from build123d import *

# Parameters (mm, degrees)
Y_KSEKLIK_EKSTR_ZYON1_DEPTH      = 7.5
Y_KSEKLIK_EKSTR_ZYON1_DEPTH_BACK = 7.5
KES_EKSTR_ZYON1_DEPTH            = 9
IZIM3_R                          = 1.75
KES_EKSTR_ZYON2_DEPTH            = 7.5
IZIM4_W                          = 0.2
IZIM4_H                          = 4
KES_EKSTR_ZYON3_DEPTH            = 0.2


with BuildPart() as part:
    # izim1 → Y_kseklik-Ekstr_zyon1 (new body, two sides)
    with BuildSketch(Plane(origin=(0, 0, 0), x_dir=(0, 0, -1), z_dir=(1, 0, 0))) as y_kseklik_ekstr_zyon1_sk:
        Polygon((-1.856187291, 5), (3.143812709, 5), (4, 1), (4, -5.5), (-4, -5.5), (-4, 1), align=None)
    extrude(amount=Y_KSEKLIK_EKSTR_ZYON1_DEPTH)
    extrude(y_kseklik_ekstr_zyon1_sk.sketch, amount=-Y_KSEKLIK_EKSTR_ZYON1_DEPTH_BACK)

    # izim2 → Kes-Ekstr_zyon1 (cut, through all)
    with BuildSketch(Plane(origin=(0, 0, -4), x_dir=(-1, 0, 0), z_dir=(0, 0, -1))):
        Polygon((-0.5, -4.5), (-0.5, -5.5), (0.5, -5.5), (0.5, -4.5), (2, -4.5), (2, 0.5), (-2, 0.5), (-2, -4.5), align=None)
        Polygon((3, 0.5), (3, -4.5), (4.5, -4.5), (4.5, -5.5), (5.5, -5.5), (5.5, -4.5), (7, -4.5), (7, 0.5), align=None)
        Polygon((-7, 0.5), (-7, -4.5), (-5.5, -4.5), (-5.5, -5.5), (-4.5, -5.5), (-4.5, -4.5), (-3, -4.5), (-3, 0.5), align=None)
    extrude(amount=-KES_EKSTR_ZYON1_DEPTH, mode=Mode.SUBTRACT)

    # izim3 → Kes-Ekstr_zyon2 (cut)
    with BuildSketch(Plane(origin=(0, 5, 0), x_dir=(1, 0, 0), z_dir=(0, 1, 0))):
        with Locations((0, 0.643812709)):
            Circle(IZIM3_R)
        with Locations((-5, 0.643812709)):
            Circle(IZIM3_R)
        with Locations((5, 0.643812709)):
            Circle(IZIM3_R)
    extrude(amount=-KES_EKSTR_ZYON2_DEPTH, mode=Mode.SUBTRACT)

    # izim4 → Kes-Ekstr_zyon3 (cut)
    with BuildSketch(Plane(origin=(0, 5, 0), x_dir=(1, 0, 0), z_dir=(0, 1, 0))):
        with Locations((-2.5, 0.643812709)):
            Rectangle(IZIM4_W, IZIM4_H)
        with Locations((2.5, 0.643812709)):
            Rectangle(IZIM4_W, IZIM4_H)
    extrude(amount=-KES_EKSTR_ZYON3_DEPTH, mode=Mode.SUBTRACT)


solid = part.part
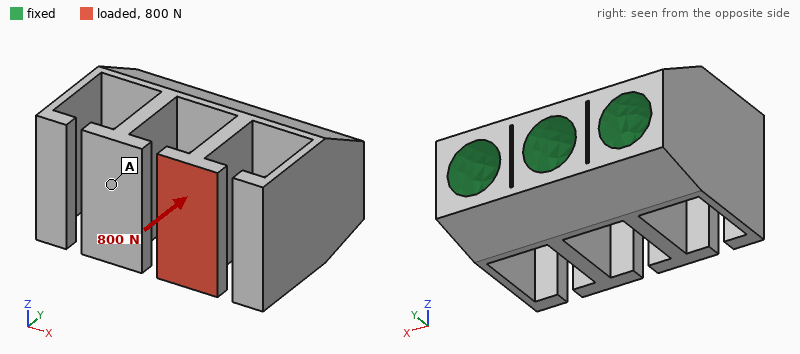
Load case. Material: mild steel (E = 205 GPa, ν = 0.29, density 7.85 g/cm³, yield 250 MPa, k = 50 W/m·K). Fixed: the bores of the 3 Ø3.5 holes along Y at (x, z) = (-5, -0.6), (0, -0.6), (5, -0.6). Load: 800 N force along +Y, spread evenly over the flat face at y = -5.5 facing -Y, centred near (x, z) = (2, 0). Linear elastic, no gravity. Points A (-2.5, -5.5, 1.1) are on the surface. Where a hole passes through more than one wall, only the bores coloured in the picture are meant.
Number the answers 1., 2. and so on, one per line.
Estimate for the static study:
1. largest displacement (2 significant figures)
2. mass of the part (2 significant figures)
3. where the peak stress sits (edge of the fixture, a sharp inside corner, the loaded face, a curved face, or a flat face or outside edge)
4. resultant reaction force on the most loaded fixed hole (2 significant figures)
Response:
1. 5.6 µm
2. 4.2 g
3. the loaded face
4. 420 N
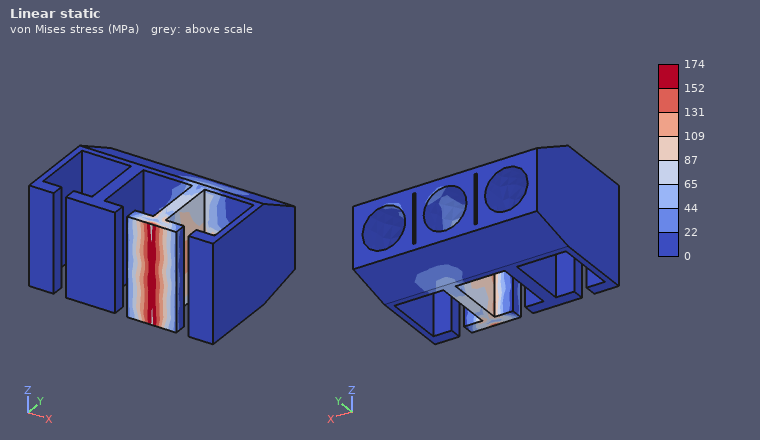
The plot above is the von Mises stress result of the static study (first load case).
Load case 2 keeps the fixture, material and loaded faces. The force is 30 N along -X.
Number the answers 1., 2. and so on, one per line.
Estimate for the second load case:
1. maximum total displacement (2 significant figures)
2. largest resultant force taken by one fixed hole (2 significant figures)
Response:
1. 19 µm
2. 75 N
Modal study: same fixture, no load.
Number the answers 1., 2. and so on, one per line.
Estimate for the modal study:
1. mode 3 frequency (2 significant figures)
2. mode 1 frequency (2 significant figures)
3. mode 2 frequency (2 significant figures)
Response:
1. 13 kHz
2. 6800 Hz
3. 6800 Hz
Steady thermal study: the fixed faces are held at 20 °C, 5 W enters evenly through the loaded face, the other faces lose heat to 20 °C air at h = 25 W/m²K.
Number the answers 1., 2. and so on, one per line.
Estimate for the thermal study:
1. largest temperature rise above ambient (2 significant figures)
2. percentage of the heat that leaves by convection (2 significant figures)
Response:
1. 77 K
2. 3.6 %
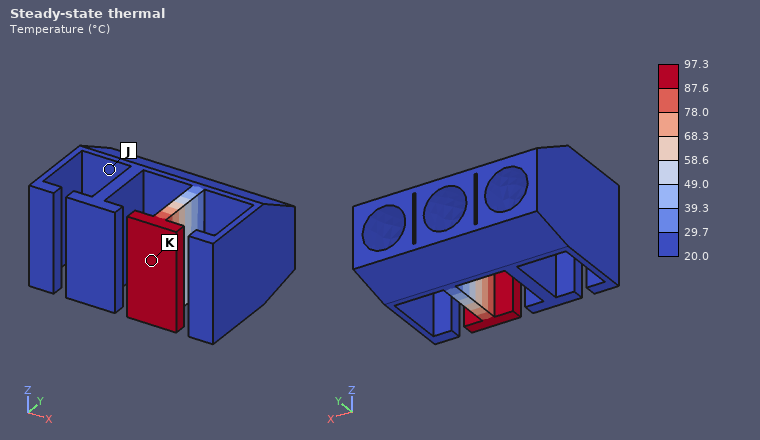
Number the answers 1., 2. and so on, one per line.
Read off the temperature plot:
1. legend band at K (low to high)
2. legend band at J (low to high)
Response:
1. 87.6 to 97.3 °C
2. 20.0 to 29.7 °C
